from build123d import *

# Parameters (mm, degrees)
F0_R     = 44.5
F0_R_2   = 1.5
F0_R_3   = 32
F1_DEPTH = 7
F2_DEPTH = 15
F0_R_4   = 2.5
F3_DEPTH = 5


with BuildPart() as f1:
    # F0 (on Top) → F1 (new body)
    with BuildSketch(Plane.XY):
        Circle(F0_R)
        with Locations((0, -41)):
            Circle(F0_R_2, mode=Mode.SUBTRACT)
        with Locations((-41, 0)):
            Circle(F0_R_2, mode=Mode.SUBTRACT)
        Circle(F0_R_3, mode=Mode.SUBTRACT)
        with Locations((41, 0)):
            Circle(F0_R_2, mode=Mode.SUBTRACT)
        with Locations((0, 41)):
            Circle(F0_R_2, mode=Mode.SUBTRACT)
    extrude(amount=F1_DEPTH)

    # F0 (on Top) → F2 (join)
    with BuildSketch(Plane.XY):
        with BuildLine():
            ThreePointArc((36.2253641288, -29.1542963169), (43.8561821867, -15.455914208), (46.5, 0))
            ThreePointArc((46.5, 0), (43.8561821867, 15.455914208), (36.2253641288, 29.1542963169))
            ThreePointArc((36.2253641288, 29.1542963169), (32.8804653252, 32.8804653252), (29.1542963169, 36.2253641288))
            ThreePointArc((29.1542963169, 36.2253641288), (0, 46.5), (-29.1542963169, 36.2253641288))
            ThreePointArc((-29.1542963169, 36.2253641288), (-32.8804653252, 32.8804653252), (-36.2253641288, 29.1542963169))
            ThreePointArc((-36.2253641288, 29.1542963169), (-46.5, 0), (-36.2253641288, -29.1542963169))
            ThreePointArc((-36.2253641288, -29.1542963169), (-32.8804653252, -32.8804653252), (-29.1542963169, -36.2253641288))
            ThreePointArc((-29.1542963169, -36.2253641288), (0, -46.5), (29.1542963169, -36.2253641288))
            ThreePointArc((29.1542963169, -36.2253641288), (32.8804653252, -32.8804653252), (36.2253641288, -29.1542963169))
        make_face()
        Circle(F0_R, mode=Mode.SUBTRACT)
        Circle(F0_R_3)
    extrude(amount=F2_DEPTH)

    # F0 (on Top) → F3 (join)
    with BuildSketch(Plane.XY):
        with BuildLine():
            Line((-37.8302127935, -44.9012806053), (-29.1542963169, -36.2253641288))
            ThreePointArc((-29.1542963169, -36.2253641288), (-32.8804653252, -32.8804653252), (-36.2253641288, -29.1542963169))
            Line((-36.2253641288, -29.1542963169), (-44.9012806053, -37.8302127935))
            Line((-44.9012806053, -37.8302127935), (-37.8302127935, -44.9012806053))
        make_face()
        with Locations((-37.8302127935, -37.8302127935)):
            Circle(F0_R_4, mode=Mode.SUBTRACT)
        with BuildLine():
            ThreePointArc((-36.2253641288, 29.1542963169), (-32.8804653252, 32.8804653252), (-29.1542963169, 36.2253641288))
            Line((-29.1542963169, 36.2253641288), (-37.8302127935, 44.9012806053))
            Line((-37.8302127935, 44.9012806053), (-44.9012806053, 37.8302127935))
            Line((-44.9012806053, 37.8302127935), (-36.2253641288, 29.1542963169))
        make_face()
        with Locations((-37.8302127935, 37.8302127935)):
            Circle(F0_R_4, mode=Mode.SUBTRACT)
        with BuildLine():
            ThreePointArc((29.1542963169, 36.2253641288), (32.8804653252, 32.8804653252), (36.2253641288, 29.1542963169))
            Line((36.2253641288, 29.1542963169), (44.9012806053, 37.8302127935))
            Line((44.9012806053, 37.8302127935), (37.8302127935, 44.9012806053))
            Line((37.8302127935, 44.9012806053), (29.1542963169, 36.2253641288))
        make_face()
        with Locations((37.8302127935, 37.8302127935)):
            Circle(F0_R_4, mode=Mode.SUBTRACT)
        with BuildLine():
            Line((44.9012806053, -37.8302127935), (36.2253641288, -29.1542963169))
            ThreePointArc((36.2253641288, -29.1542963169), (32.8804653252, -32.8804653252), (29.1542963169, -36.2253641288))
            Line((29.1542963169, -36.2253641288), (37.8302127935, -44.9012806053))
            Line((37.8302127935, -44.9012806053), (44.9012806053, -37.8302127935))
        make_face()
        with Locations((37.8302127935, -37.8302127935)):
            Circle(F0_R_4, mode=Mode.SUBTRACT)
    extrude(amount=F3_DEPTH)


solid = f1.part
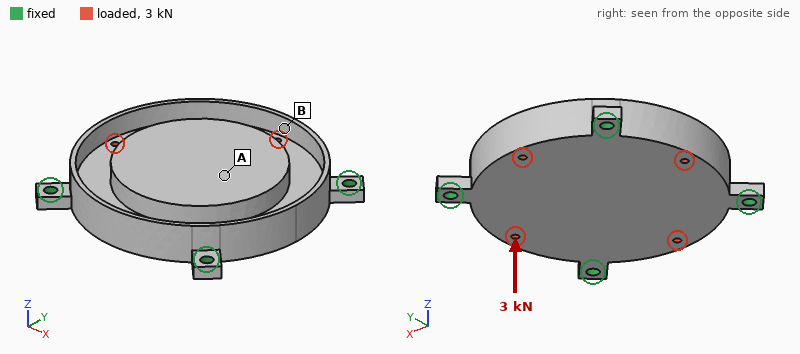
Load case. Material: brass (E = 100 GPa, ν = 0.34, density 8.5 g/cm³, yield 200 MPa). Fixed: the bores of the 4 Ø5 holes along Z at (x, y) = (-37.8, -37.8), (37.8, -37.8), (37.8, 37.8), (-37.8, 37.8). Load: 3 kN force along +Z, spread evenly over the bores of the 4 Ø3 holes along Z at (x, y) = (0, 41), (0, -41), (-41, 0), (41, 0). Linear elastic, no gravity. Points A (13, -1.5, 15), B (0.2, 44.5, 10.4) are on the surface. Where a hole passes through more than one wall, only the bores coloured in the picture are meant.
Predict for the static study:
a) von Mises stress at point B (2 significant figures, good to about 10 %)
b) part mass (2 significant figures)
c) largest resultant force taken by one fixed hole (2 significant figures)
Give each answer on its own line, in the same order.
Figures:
26 MPa
680 g
900 N
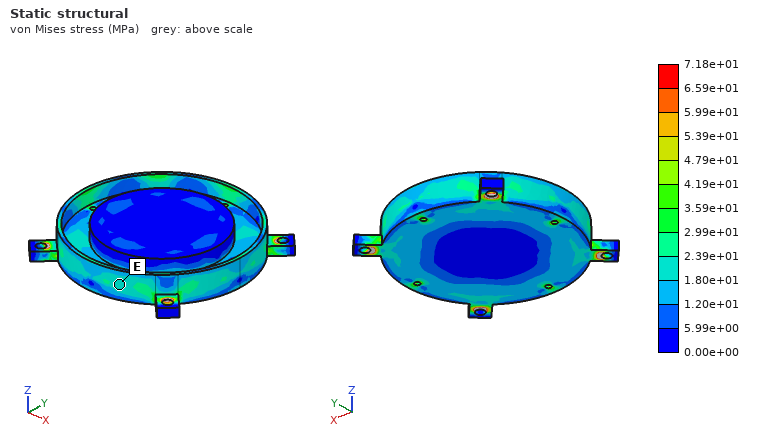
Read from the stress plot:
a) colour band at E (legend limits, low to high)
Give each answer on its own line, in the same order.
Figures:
1.80e+01 to 2.39e+01 MPa
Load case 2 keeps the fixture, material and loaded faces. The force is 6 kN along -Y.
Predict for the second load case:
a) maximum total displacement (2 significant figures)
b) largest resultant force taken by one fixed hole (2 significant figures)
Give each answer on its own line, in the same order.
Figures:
10 µm
1.6 kN
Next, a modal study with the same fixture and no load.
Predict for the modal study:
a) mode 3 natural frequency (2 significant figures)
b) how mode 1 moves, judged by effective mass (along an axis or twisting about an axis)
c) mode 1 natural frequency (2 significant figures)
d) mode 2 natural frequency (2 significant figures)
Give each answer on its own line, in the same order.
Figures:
3700 Hz
along Z
2400 Hz
3700 Hz
